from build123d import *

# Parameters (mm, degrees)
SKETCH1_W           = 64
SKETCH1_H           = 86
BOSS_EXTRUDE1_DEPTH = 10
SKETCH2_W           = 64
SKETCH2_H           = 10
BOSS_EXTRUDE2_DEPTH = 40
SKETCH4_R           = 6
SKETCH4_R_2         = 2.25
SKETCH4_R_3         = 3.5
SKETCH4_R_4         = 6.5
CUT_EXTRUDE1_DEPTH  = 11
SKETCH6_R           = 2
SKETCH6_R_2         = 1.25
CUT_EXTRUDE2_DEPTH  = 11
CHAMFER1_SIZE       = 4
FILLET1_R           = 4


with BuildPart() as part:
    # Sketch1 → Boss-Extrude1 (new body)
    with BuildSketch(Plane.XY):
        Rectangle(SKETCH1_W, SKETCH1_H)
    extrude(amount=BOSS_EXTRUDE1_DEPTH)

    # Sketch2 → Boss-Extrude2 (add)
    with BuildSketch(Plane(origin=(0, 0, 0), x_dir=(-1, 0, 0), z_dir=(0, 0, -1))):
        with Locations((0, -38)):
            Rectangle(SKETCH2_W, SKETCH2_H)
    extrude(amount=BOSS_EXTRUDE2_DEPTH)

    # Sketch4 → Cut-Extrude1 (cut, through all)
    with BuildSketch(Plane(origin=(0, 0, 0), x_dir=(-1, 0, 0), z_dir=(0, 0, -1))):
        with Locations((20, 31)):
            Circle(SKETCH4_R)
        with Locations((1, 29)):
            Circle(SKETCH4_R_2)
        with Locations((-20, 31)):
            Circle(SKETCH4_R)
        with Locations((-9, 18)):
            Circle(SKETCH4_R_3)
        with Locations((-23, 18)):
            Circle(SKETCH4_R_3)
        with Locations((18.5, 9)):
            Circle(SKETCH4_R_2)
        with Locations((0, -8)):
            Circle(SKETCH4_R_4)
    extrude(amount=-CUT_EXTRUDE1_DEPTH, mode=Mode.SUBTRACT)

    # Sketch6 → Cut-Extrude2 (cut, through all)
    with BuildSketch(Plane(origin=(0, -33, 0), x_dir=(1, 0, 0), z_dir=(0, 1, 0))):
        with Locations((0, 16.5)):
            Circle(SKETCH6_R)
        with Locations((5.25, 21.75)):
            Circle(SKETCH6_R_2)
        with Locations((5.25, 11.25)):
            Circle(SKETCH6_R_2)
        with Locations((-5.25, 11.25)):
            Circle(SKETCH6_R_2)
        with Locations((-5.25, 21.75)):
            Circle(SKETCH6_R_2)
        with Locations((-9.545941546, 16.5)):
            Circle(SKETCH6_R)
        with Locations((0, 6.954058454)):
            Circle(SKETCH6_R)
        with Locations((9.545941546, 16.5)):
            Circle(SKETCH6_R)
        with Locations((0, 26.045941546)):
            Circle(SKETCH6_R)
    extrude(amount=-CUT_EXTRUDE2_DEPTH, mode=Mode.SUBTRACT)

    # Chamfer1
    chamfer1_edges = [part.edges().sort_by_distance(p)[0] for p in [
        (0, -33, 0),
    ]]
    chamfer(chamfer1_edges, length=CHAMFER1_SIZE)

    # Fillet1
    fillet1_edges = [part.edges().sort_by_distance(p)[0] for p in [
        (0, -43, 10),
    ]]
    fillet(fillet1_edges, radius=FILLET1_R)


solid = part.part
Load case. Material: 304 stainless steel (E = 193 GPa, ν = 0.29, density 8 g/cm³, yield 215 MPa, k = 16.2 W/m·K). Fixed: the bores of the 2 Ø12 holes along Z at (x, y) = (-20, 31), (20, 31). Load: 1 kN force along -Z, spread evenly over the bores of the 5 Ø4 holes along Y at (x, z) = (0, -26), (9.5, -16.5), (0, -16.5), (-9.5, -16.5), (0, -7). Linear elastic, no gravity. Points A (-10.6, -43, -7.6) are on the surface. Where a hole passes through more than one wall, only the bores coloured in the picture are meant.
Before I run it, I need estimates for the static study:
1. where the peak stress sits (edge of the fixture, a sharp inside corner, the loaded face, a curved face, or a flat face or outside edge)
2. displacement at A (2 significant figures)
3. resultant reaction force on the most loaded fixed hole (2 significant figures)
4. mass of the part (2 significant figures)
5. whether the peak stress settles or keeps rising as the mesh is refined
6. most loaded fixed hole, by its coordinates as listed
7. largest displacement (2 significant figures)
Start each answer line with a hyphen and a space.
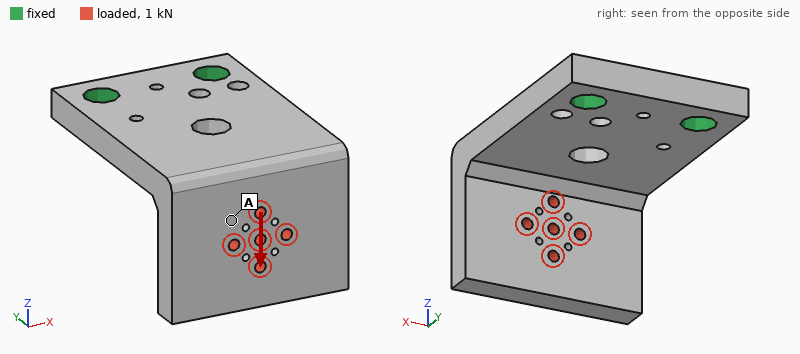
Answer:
- a sharp inside corner
- 0.12 mm
- 560 N
- 600 g
- keeps rising
- (-20, 31)
- 0.17 mm
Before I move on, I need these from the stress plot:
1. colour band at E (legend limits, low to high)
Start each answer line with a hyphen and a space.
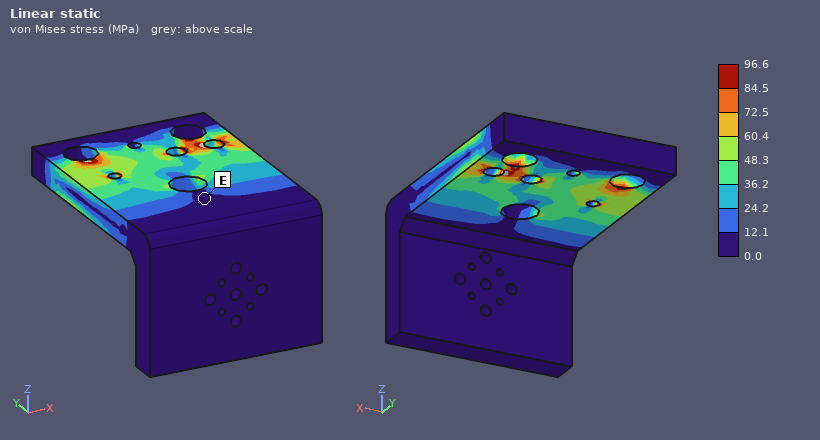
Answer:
- 0.0 to 12.1 MPa
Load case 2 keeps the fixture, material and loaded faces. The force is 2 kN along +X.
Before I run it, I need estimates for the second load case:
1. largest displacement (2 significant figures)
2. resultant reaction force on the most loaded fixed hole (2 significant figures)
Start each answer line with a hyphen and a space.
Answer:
- 84 µm
- 3.2 kN
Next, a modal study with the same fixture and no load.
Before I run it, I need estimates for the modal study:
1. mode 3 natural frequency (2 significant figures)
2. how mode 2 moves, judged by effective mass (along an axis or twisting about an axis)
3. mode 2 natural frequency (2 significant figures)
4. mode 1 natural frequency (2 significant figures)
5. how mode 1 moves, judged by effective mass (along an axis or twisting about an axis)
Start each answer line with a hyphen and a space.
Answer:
- 2900 Hz
- along X
- 1700 Hz
- 770 Hz
- along Z
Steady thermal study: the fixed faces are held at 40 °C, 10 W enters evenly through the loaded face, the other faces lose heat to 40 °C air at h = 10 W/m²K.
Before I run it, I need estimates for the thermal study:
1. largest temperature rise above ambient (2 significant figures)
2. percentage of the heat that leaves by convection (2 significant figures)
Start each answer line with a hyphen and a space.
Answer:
- 57 K
- 52 %
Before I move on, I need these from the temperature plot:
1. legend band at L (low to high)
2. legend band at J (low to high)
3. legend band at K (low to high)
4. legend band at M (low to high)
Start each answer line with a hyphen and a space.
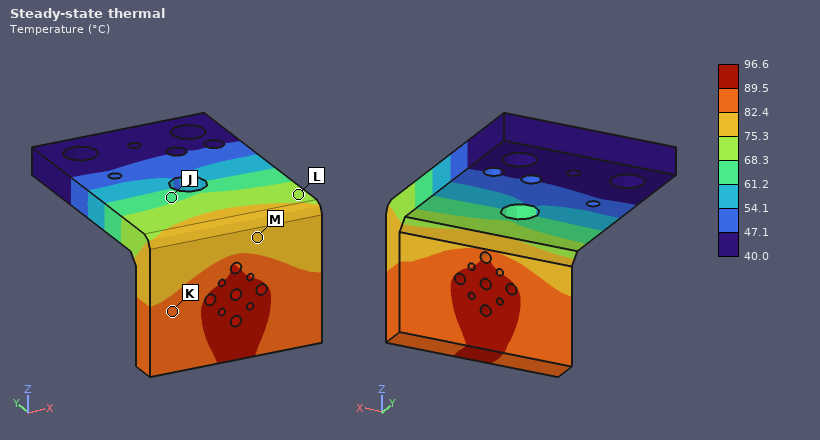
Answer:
- 68.3 to 75.3 °C
- 61.2 to 68.3 °C
- 82.4 to 89.5 °C
- 75.3 to 82.4 °C
